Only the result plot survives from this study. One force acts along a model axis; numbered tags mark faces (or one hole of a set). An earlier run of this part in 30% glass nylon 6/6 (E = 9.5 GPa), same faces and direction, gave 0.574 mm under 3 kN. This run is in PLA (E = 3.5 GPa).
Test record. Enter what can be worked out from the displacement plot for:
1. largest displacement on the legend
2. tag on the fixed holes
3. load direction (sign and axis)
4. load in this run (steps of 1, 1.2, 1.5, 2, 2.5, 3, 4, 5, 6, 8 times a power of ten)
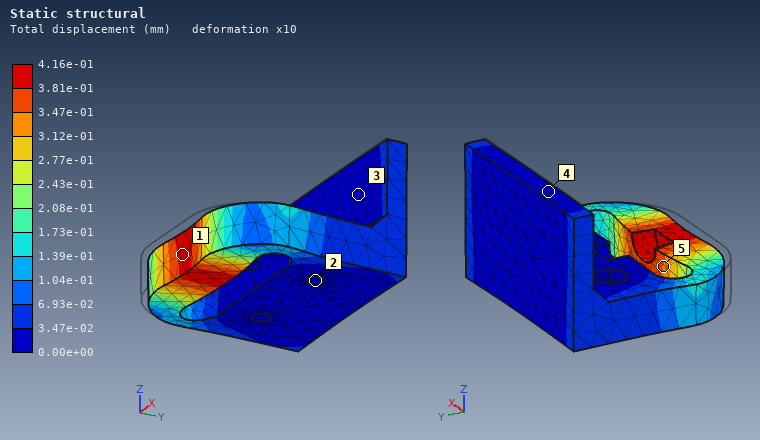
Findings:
4.16e-01 mm
2
+Y
800 N
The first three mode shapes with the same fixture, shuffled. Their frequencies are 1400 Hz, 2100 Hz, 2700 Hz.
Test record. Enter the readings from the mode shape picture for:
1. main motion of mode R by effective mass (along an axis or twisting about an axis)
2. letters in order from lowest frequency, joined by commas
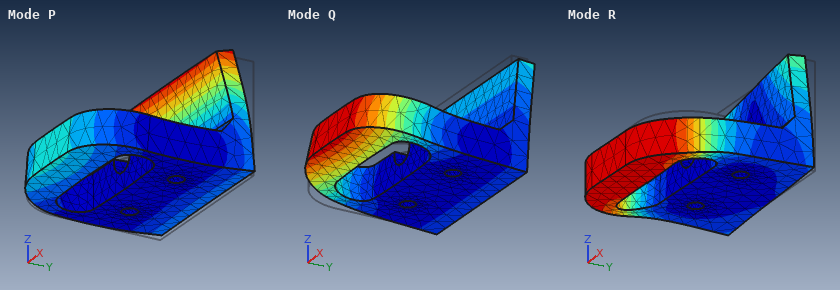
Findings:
along X
Q, P, R
